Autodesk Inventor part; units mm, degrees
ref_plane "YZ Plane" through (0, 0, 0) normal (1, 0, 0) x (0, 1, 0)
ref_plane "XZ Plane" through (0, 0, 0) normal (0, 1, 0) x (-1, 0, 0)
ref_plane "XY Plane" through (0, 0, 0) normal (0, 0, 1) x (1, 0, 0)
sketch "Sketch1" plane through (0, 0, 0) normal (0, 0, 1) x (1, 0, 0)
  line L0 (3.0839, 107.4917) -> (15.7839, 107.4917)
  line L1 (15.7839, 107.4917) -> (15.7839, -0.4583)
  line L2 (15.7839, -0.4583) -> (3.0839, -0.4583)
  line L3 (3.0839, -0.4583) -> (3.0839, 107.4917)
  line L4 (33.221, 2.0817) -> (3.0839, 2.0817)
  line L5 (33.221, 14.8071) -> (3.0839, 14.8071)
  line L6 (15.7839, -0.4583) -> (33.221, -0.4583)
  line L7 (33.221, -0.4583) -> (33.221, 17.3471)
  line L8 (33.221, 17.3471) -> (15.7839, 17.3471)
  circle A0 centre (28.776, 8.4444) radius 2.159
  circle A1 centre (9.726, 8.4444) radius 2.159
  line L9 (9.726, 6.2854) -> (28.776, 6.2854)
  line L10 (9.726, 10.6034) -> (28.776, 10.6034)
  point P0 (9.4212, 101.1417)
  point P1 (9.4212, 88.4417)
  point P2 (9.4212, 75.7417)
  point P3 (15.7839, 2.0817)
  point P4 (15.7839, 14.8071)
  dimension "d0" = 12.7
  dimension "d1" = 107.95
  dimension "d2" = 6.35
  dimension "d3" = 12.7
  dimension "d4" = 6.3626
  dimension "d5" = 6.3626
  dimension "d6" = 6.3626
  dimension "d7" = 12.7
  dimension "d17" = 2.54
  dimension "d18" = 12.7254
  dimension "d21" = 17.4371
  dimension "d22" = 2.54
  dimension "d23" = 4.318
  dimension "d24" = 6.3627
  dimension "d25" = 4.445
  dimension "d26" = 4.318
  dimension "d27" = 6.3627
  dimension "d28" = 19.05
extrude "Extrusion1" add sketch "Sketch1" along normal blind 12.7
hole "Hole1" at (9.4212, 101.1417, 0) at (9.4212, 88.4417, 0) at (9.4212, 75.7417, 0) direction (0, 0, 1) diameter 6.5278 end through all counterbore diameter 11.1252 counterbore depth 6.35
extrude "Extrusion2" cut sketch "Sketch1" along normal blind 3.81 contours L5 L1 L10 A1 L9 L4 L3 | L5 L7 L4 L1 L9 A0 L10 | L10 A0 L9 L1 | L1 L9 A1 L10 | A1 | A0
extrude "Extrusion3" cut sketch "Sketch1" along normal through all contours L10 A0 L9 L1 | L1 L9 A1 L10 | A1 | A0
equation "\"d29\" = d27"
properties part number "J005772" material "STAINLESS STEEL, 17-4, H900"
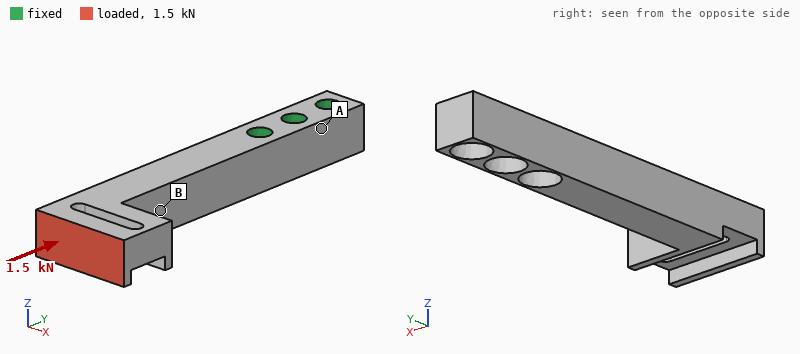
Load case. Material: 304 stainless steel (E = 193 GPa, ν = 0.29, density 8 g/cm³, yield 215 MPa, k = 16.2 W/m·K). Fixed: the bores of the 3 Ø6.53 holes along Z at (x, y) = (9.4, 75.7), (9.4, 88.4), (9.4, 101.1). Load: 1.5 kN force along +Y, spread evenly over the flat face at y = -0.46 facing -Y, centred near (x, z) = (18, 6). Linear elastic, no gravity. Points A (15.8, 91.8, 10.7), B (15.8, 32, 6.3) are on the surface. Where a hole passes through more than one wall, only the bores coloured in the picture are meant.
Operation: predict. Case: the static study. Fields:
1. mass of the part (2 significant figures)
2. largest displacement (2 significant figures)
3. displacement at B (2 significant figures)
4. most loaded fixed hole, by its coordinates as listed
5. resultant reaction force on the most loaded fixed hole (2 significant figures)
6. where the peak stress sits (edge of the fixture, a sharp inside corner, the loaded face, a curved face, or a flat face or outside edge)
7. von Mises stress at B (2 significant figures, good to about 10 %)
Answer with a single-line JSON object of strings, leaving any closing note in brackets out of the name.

{"mass of the part": "130 g", "largest displacement": "0.15 mm", "displacement at B": "0.040 mm", "most loaded fixed hole, by its coordinates as listed": "(9.4, 75.7)", "resultant reaction force on the most loaded fixed hole": "1.3 kN", "where the peak stress sits": "a curved face", "von Mises stress at B": "46 MPa"}
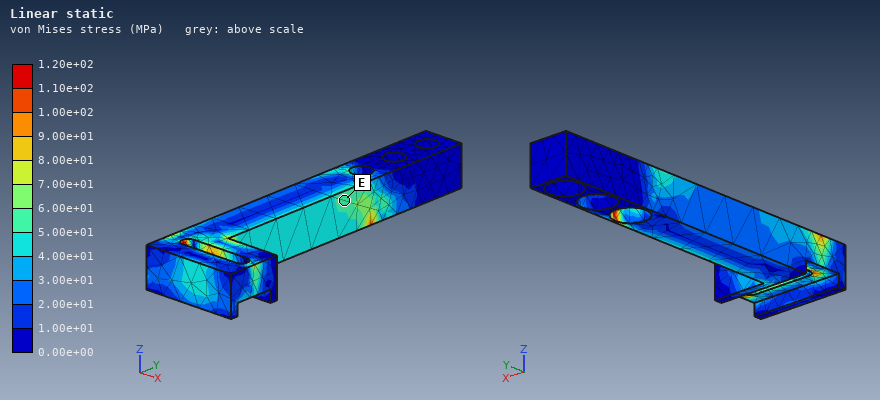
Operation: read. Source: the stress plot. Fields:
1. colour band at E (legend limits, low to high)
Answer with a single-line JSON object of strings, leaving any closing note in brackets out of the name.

{"colour band at E": "5.00e+01 to 6.00e+01 MPa"}
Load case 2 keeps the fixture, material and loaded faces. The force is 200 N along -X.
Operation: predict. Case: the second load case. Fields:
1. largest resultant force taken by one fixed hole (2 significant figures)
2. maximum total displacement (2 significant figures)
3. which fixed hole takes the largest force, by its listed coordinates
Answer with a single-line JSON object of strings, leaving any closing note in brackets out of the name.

{"largest resultant force taken by one fixed hole": "480 N", "maximum total displacement": "98 µm", "which fixed hole takes the largest force, by its listed coordinates": "(9.4, 75.7)"}
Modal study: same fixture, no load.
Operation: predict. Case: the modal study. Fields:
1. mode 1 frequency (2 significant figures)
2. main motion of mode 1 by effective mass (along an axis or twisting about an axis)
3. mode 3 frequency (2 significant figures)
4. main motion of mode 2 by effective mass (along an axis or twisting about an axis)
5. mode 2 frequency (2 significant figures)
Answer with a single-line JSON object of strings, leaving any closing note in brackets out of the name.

{"mode 1 frequency": "1100 Hz", "main motion of mode 1 by effective mass": "along Z", "mode 3 frequency": "4400 Hz", "main motion of mode 2 by effective mass": "along X", "mode 2 frequency": "1300 Hz"}
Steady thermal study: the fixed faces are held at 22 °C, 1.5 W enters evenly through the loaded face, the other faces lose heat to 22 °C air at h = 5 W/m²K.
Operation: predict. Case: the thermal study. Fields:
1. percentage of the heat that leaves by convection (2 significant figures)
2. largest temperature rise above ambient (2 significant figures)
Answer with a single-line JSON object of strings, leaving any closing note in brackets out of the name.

{"percentage of the heat that leaves by convection": "36 %", "largest temperature rise above ambient": "43 K"}
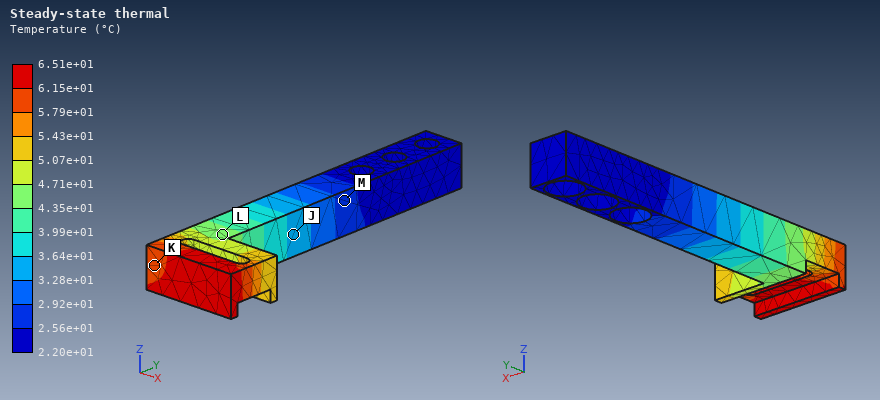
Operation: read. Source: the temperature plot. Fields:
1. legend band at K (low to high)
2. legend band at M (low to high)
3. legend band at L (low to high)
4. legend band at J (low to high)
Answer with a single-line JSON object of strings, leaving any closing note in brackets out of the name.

{"legend band at K": "5.79e+01 to 6.15e+01 °C", "legend band at M": "2.56e+01 to 2.92e+01 °C", "legend band at L": "4.35e+01 to 4.71e+01 °C", "legend band at J": "3.28e+01 to 3.64e+01 °C"}
